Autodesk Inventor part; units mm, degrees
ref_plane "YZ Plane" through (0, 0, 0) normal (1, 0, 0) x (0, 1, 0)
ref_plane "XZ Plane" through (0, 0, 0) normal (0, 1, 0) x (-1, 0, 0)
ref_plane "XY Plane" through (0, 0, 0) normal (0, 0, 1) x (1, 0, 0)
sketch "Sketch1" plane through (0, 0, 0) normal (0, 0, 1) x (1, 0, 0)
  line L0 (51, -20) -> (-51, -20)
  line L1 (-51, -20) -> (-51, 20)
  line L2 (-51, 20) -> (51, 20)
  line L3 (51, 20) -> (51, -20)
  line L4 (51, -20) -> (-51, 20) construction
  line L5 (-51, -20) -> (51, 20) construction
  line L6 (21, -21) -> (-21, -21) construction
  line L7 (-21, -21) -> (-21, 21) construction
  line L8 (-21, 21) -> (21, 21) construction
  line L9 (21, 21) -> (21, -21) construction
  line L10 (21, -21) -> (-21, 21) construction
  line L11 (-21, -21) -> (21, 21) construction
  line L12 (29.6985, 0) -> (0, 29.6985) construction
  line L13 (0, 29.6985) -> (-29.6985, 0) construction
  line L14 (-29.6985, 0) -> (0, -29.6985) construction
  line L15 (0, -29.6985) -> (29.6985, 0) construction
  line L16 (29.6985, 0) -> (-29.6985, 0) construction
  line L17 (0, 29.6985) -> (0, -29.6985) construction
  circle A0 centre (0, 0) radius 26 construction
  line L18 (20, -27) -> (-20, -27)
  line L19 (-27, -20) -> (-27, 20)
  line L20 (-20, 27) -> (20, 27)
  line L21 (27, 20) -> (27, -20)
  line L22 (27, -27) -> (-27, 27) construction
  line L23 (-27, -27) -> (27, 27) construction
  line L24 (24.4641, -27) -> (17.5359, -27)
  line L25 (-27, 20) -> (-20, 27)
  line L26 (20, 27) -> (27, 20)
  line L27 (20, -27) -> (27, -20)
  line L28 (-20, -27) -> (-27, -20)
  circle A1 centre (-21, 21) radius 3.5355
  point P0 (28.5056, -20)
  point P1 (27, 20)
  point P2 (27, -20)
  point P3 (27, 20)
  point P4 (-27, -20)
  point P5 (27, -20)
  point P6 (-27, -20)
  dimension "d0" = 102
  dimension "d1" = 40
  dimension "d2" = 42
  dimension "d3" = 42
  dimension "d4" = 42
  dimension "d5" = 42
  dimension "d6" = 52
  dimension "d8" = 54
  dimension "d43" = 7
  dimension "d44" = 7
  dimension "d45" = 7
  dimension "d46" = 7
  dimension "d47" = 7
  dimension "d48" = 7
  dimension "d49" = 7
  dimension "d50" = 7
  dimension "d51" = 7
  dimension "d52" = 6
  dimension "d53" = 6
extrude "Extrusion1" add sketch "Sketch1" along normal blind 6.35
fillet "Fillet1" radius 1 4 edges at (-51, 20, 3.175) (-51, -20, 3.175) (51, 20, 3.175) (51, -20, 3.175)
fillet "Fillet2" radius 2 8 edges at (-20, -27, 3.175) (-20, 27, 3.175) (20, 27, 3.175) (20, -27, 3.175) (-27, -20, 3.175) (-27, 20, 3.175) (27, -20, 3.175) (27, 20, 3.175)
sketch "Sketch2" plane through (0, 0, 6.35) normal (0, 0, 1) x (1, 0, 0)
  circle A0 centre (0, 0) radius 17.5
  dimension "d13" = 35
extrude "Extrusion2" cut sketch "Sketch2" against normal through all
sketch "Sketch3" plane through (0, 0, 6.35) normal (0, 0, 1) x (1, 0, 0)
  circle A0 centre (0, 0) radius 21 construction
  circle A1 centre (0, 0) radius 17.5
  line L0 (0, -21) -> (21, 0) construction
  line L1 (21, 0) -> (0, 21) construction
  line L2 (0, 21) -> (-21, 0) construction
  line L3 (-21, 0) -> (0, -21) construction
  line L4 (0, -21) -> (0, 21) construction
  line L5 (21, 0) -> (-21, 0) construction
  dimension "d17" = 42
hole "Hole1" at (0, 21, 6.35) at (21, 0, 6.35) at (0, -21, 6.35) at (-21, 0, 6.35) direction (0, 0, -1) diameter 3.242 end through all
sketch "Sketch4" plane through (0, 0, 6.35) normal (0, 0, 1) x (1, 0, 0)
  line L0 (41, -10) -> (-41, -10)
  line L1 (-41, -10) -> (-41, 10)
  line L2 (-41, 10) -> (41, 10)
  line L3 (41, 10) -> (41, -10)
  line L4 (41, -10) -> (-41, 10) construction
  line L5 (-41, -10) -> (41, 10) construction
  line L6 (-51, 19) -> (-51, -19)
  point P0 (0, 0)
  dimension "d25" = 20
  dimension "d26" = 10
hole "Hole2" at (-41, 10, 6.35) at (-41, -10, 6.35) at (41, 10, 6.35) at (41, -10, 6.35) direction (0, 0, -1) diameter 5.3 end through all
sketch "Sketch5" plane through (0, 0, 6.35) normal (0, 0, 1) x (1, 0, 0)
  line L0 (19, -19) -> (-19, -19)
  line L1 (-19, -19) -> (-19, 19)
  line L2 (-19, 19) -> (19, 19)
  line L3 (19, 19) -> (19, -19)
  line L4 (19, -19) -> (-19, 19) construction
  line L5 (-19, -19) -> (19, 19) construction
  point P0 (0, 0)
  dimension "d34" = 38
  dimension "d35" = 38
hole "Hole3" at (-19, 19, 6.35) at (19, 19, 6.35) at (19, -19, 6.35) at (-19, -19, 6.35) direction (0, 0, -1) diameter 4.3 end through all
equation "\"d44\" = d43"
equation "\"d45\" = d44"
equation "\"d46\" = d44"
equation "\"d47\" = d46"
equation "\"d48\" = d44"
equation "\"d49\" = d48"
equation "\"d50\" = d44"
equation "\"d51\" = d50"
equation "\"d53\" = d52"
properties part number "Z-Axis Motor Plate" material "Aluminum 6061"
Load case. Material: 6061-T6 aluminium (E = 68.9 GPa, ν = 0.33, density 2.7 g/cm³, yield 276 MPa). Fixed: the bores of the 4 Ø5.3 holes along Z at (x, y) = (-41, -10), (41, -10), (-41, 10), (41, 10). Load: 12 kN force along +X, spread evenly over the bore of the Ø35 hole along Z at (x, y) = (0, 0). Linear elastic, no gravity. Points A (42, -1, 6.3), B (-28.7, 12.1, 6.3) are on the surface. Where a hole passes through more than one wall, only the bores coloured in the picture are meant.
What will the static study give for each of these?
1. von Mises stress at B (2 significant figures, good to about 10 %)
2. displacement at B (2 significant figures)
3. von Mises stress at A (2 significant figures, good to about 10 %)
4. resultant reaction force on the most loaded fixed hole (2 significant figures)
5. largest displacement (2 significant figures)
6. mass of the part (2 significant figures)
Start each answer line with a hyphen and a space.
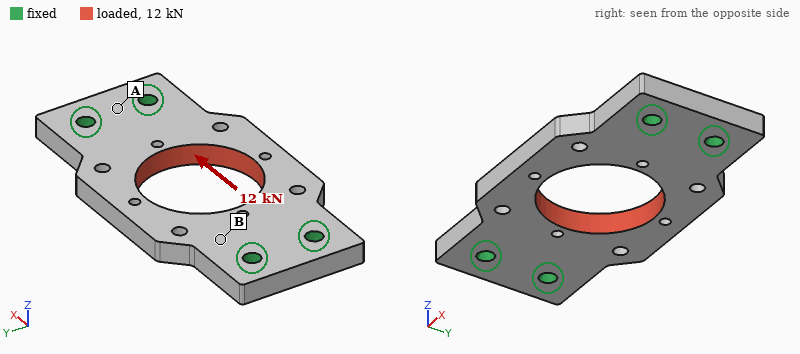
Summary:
- 27 MPa
- 5.3 µm
- 7.7 MPa
- 3.0 kN
- 18 µm
- 62 g
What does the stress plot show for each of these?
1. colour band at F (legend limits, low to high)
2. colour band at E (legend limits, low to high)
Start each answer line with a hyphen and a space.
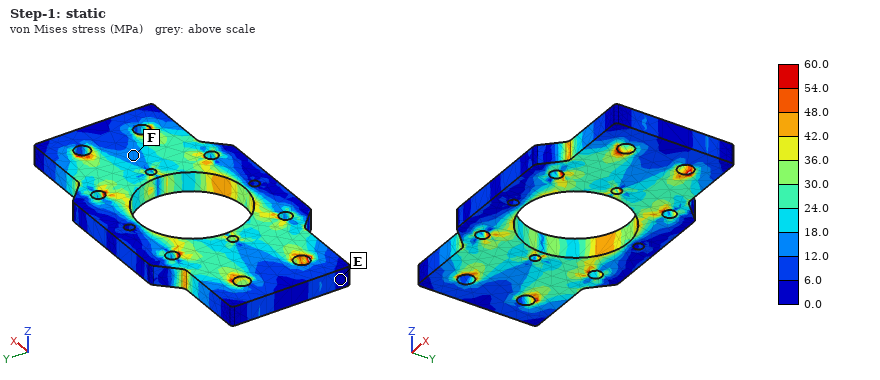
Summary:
- 12.0 to 18.0 MPa
- 0.0 to 6.0 MPa
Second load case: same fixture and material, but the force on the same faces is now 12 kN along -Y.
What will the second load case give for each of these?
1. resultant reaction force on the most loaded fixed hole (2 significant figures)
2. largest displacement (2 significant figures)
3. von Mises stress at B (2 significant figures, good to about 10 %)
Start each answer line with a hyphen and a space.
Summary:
- 3.9 kN
- 53 µm
- 34 MPa
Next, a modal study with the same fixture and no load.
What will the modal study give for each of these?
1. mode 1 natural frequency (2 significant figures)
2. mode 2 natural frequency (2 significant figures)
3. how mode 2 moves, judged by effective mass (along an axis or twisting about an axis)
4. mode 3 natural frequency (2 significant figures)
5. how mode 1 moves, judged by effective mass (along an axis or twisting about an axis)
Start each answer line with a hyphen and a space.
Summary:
- 4900 Hz
- 5200 Hz
- twisting about X
- 11 kHz
- along Z
